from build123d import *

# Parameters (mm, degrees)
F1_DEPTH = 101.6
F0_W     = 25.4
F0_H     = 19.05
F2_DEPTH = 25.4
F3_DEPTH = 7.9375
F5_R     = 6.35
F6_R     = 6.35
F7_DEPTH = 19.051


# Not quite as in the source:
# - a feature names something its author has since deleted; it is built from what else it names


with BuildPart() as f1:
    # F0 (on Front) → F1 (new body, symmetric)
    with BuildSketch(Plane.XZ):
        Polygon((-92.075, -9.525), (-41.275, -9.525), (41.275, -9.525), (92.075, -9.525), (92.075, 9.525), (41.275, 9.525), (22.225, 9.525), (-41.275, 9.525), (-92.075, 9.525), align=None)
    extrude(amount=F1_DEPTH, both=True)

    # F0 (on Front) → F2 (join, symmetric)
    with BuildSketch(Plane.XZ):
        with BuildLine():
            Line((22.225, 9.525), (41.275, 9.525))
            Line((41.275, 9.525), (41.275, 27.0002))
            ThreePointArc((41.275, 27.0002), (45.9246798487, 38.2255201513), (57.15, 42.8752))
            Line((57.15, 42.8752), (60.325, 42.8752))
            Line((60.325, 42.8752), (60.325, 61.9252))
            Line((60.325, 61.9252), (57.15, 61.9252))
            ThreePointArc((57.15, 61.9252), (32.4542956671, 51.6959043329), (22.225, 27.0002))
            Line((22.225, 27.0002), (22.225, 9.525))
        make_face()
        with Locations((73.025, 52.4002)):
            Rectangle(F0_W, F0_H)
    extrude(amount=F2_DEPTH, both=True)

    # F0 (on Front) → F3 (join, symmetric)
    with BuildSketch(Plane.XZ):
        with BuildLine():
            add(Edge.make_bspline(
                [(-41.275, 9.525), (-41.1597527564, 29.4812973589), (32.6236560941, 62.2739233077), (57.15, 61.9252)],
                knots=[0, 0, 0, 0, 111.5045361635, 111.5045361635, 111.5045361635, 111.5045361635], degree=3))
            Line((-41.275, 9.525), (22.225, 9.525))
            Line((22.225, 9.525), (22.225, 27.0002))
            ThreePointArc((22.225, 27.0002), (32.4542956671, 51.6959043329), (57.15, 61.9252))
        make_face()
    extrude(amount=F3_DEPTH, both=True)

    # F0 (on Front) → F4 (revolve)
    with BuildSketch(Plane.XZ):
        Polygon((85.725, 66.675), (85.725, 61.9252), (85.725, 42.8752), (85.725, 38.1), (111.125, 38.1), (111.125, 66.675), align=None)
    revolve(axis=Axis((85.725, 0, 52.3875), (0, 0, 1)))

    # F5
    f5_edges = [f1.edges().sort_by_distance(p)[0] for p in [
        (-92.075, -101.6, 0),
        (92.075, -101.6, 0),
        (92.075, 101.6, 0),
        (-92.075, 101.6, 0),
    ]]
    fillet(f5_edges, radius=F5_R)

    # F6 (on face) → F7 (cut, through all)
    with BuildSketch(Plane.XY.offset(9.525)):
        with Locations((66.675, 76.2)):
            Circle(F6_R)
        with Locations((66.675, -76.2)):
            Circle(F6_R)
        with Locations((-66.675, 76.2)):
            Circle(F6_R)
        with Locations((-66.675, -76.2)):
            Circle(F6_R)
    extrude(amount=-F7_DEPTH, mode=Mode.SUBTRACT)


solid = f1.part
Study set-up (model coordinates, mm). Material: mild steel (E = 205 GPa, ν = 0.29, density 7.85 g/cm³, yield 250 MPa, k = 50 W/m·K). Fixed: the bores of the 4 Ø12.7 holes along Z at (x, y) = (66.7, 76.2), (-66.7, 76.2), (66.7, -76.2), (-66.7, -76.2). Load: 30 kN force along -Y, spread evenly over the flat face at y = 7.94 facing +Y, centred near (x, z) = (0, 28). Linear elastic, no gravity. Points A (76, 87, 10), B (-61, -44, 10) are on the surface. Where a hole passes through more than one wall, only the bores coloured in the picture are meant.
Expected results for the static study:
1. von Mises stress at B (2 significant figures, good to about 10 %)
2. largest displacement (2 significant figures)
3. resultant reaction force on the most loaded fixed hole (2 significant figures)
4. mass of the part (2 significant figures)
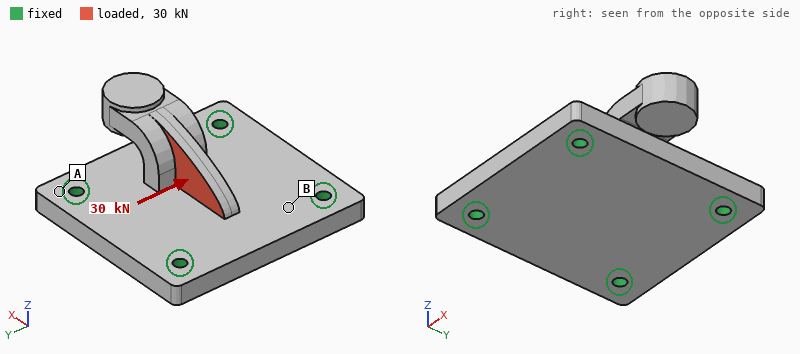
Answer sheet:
13 MPa
47 µm
9.5 kN
6.7 kg
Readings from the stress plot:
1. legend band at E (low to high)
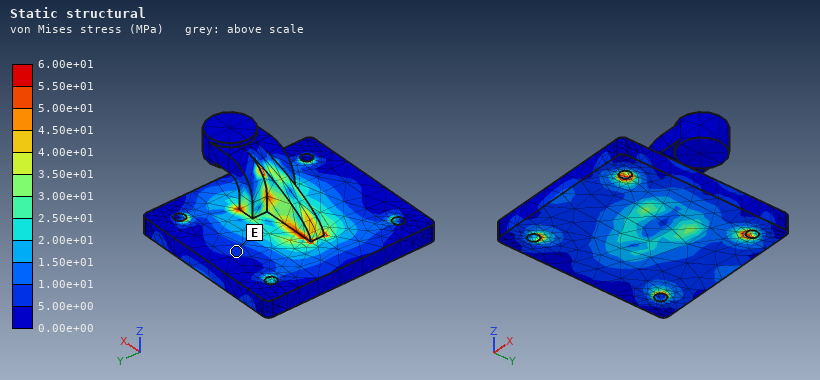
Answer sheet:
5.00e+00 to 1.00e+01 MPa
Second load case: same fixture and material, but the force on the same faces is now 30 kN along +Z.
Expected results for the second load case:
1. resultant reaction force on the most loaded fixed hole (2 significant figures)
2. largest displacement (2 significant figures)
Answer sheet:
8.9 kN
58 µm
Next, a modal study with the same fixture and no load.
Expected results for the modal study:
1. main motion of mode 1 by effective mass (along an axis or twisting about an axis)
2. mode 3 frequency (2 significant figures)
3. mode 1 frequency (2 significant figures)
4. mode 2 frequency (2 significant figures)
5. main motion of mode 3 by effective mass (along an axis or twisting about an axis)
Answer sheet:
along Z
2800 Hz
1600 Hz
1900 Hz
along Z
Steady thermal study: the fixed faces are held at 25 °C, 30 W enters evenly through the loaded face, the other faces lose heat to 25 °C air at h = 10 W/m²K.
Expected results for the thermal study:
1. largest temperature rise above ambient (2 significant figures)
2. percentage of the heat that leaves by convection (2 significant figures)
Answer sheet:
19 K
17 %
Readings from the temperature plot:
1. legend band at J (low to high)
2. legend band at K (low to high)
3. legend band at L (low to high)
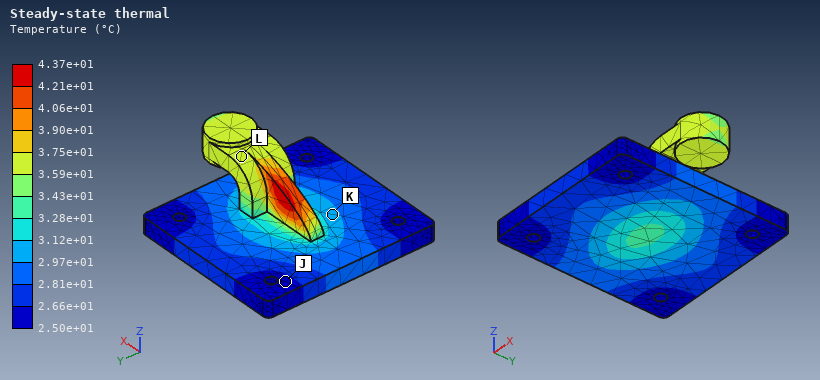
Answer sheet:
2.50e+01 to 2.66e+01 °C
2.97e+01 to 3.12e+01 °C
3.59e+01 to 3.75e+01 °C
